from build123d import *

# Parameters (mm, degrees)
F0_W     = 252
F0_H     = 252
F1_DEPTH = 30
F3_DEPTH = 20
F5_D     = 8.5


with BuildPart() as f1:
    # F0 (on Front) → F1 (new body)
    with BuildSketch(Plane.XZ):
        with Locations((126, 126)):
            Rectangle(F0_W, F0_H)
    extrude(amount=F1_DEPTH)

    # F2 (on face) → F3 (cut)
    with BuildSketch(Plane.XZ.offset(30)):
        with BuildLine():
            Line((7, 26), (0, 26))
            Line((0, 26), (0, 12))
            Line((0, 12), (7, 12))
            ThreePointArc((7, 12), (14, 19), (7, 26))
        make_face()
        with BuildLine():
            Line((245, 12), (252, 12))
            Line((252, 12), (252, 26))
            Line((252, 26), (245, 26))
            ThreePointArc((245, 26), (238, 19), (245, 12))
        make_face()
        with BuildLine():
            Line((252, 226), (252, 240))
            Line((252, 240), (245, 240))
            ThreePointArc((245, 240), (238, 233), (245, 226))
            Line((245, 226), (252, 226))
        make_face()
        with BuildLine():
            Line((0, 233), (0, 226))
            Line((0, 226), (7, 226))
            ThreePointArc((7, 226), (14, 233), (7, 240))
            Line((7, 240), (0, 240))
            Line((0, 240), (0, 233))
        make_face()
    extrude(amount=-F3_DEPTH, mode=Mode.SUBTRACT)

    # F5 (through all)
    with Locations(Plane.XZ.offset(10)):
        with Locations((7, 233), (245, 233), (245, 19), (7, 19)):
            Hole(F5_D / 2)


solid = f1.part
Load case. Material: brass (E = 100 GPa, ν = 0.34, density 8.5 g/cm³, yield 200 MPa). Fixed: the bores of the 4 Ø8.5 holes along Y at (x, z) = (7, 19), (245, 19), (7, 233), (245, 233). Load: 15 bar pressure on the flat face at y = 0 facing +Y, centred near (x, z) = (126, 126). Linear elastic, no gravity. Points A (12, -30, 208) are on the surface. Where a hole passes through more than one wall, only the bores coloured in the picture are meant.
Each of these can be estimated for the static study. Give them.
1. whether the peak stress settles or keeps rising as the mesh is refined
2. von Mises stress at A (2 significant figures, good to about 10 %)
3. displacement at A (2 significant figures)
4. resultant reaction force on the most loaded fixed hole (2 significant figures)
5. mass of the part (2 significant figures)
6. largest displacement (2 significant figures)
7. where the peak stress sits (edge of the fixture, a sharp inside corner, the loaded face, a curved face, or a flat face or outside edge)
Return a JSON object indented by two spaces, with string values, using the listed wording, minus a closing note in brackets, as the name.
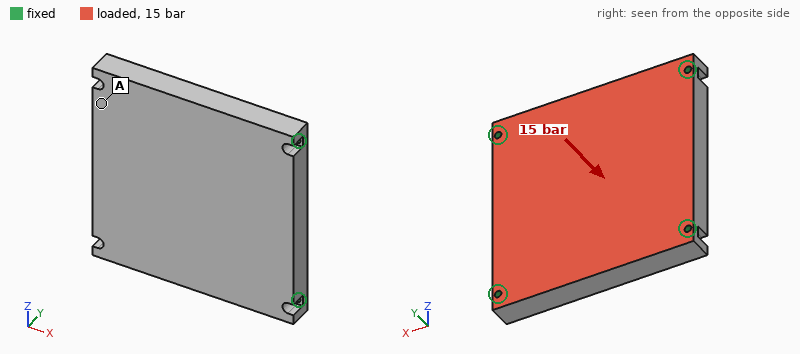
{
  "whether the peak stress settles or keeps rising as the mesh is refined": "keeps rising",
  "von Mises stress at A": "27 MPa",
  "displacement at A": "0.078 mm",
  "resultant reaction force on the most loaded fixed hole": "37 kN",
  "mass of the part": "16 kg",
  "largest displacement": "0.27 mm",
  "where the peak stress sits": "edge of the fixture"
}
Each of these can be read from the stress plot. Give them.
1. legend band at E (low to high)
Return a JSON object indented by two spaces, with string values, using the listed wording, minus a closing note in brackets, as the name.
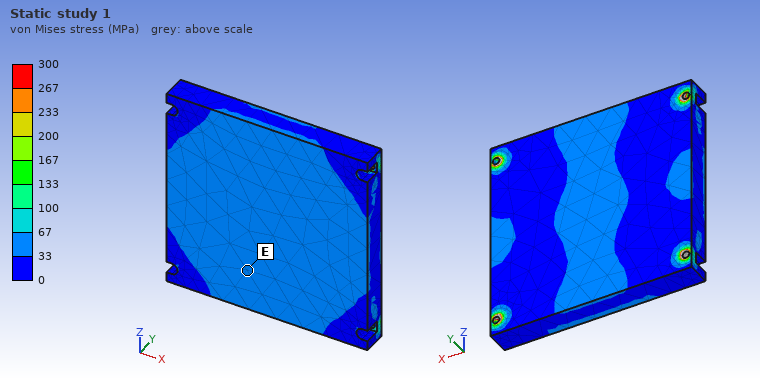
{
  "legend band at E": "33 to 67 MPa"
}
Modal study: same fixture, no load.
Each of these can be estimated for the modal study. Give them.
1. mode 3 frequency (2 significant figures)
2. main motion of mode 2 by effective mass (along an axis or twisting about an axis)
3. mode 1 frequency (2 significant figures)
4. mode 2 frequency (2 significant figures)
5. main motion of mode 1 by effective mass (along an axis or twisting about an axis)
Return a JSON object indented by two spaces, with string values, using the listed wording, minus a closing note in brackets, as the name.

{
  "mode 3 frequency": "1600 Hz",
  "main motion of mode 2 by effective mass": "twisting about X",
  "mode 1 frequency": "860 Hz",
  "mode 2 frequency": "1400 Hz",
  "main motion of mode 1 by effective mass": "along Y"
}
